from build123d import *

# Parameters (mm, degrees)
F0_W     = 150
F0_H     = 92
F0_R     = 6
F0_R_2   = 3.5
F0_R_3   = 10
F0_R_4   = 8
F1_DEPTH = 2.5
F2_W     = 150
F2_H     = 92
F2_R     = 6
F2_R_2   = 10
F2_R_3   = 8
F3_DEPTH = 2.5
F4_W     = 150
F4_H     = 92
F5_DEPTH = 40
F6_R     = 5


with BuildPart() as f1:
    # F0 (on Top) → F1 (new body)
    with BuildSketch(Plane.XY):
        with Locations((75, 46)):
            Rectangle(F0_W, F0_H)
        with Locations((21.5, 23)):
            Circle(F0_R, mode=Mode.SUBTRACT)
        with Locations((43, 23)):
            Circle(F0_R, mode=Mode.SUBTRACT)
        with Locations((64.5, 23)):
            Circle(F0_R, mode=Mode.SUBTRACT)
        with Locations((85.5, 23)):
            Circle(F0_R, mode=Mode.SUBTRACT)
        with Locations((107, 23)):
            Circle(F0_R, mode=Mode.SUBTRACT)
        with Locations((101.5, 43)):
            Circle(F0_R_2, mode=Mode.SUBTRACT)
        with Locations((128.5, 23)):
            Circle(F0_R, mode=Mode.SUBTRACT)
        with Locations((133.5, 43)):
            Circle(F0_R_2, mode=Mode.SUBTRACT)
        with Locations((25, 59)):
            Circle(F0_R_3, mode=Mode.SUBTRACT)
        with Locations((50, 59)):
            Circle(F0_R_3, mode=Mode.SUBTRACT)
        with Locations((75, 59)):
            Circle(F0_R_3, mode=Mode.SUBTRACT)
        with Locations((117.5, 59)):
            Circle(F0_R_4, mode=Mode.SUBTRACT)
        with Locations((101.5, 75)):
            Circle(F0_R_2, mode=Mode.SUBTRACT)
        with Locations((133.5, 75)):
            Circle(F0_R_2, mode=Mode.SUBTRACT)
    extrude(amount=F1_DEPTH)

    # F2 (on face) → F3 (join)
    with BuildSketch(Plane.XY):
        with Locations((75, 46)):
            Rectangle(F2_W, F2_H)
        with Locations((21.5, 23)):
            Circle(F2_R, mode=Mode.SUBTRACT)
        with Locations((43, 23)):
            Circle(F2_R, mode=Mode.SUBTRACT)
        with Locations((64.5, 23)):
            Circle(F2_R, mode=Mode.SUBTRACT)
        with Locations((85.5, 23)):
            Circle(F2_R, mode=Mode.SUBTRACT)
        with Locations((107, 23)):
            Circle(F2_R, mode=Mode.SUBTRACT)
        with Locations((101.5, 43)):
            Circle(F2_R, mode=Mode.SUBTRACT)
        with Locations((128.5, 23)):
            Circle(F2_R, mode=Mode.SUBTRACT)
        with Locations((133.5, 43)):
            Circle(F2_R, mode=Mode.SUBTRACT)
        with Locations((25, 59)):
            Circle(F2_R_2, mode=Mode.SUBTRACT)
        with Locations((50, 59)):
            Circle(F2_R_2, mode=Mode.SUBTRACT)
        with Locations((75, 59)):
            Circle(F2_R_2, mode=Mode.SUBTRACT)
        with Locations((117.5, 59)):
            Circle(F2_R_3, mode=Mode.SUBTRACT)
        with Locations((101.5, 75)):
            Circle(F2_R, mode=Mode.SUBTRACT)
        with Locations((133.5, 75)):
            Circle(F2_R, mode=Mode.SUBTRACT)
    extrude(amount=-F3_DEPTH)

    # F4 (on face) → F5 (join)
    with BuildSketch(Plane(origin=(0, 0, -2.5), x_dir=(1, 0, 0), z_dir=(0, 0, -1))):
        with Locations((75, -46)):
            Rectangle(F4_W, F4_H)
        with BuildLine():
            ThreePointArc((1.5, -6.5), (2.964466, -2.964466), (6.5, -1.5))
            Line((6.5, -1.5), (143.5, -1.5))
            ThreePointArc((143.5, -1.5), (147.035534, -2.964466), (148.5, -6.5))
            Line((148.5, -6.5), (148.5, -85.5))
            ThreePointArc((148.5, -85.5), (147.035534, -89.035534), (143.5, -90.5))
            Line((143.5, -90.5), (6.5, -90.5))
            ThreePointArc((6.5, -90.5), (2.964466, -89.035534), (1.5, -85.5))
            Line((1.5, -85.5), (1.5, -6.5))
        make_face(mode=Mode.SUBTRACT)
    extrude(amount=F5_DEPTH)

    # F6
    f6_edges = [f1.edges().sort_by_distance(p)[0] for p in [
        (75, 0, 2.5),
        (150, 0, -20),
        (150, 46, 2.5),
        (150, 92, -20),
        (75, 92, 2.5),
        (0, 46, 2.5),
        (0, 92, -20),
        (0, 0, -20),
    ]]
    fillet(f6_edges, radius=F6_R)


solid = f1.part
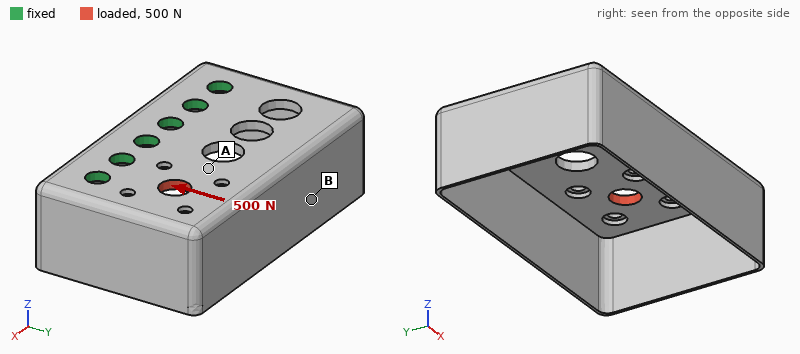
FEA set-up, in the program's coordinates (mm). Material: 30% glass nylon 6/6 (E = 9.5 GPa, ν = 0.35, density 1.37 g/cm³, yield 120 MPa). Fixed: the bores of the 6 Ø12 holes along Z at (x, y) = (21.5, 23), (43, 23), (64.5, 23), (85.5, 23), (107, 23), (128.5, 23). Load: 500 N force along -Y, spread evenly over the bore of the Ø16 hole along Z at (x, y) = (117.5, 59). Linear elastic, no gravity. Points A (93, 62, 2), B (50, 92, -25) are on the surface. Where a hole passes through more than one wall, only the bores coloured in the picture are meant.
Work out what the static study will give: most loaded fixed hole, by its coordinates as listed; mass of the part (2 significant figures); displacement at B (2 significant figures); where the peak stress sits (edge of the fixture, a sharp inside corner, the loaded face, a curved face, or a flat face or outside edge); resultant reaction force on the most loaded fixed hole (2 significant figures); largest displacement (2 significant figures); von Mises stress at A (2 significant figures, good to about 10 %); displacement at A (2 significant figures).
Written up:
(128.5, 23)
120 g
4.0 µm
a curved face
280 N
13 µm
0.67 MPa
3.9 µm
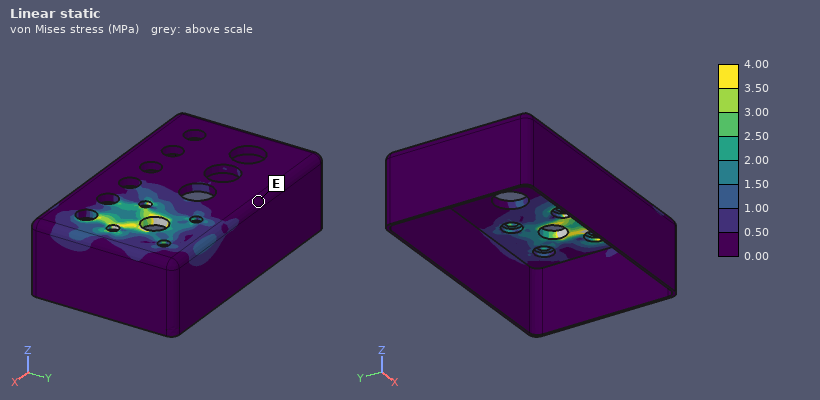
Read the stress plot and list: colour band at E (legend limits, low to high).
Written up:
0.00 to 0.50 MPa
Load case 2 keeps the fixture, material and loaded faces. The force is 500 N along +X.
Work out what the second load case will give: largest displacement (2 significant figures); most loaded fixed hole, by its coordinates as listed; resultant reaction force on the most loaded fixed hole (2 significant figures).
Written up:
22 µm
(128.5, 23)
270 N
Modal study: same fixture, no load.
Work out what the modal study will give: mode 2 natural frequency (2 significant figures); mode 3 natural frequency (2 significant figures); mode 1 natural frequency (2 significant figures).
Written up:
490 Hz
570 Hz
450 Hz
